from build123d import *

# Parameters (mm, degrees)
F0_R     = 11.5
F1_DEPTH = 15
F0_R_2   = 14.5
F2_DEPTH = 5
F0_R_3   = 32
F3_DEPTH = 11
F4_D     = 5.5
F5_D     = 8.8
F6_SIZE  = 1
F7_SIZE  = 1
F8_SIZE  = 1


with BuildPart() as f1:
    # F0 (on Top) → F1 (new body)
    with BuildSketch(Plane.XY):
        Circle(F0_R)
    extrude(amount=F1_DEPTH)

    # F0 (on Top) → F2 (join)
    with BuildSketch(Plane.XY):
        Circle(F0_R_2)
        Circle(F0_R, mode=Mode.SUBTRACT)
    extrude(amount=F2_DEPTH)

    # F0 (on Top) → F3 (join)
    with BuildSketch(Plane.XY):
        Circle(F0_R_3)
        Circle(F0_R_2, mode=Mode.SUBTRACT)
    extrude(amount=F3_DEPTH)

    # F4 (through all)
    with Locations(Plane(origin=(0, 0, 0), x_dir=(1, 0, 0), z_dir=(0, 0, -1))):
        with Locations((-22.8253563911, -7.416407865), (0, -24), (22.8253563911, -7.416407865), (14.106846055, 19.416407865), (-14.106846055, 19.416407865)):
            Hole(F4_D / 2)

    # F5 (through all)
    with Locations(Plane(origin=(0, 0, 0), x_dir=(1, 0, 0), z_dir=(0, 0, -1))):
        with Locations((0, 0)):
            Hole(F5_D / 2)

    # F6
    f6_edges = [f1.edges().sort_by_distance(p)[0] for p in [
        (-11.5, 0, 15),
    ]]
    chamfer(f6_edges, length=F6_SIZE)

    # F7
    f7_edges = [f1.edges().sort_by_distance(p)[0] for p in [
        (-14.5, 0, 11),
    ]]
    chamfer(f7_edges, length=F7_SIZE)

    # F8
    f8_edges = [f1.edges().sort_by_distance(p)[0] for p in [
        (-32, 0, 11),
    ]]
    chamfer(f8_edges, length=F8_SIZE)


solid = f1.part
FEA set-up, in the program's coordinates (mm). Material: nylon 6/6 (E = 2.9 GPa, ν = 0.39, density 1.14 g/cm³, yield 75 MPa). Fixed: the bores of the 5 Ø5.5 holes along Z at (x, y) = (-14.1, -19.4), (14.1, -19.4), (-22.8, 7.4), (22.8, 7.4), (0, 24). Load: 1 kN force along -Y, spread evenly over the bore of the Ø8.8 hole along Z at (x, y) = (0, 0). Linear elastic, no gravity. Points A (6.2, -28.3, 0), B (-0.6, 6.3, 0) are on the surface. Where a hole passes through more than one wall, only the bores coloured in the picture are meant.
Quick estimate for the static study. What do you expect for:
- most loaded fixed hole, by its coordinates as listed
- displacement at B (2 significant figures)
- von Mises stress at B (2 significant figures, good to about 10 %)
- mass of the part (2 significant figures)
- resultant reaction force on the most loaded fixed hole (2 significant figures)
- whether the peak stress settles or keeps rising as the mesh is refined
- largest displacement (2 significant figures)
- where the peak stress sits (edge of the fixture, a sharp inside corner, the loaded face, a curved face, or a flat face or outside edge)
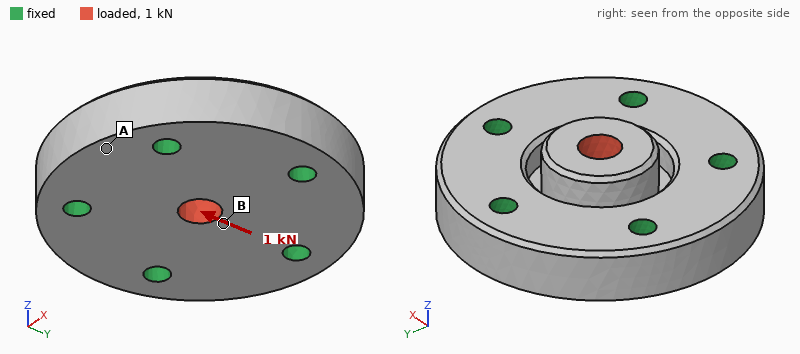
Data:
(0, 24)
21 µm
2.3 MPa
38 g
300 N
keeps rising
63 µm
edge of the fixture
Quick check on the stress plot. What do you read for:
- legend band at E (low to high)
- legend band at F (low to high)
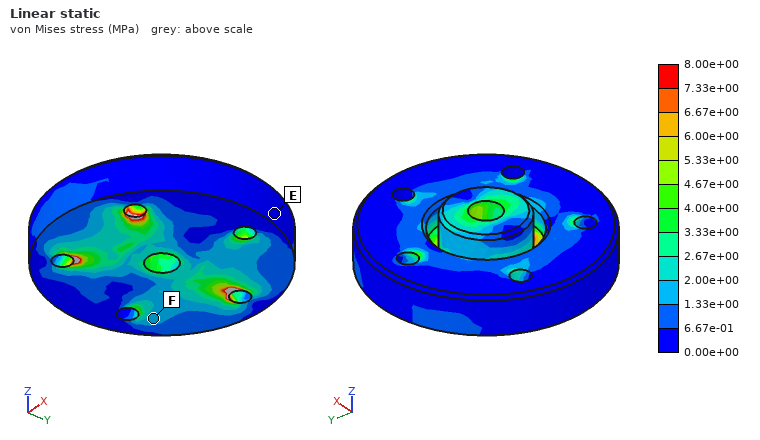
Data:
0.00e+00 to 6.67e-01 MPa
1.33e+00 to 2.00e+00 MPa
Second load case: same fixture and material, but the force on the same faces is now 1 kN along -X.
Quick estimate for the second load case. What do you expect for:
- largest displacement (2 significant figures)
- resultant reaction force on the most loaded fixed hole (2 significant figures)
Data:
63 µm
290 N
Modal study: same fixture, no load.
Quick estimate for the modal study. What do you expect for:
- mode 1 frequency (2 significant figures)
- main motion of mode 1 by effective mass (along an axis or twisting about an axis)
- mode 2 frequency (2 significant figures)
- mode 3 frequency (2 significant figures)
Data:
8000 Hz
along Z
8800 Hz
8800 Hz
